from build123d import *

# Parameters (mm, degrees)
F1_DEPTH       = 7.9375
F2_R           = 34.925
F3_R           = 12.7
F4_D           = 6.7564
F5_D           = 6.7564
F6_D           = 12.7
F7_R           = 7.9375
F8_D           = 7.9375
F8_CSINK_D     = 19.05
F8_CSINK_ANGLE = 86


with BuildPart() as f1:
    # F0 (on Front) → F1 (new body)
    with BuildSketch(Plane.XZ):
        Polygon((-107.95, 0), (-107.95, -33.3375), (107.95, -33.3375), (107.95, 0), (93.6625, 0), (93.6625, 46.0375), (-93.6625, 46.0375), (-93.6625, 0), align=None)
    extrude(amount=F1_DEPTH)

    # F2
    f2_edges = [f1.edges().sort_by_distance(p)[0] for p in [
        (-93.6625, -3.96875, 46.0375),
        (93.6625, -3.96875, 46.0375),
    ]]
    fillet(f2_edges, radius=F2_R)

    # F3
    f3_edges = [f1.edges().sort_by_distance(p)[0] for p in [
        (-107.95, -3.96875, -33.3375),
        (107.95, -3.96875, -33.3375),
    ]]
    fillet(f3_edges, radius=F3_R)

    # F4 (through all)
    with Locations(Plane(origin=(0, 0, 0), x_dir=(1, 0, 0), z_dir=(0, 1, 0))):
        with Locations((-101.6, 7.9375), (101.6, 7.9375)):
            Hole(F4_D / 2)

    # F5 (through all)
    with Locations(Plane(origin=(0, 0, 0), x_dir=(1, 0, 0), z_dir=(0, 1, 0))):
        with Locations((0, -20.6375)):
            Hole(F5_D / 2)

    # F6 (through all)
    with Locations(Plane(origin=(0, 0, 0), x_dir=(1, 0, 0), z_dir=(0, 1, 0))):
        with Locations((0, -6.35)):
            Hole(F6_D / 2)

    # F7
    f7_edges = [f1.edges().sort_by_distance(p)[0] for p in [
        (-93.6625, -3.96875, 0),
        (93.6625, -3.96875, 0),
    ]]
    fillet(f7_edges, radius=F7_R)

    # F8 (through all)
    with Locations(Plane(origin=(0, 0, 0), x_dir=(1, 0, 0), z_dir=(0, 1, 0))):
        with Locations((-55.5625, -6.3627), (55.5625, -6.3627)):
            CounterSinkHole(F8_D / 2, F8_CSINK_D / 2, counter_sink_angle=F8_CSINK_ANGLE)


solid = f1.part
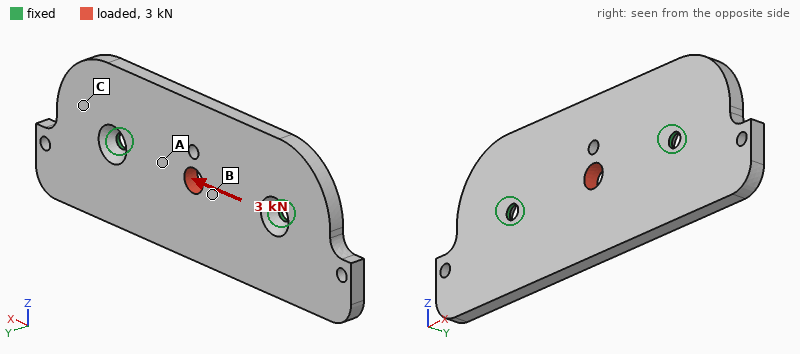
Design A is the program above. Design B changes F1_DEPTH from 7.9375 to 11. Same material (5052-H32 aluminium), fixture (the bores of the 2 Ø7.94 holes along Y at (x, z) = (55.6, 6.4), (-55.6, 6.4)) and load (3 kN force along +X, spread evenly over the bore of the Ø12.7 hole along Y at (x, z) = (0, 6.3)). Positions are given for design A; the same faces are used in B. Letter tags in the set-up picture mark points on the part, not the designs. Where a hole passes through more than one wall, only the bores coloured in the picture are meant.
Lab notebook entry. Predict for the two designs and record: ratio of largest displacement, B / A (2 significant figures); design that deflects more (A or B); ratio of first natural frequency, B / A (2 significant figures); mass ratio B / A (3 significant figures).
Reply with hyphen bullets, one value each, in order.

- 0.32
- A
- 1.6
- 1.39
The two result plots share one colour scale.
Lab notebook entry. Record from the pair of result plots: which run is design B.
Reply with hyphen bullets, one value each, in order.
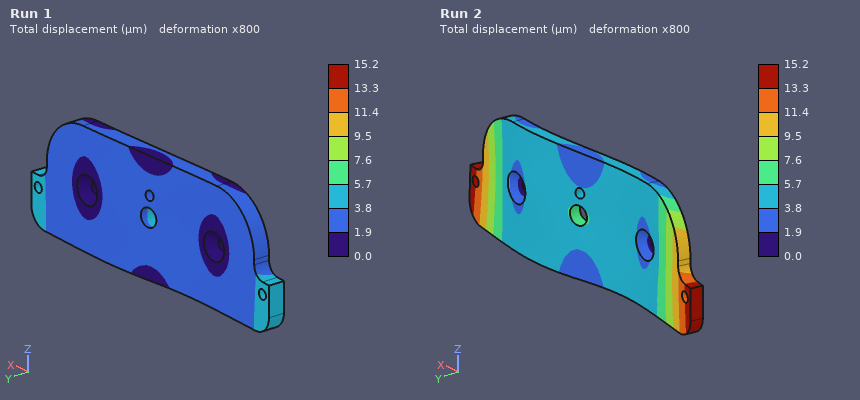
- Run 1
